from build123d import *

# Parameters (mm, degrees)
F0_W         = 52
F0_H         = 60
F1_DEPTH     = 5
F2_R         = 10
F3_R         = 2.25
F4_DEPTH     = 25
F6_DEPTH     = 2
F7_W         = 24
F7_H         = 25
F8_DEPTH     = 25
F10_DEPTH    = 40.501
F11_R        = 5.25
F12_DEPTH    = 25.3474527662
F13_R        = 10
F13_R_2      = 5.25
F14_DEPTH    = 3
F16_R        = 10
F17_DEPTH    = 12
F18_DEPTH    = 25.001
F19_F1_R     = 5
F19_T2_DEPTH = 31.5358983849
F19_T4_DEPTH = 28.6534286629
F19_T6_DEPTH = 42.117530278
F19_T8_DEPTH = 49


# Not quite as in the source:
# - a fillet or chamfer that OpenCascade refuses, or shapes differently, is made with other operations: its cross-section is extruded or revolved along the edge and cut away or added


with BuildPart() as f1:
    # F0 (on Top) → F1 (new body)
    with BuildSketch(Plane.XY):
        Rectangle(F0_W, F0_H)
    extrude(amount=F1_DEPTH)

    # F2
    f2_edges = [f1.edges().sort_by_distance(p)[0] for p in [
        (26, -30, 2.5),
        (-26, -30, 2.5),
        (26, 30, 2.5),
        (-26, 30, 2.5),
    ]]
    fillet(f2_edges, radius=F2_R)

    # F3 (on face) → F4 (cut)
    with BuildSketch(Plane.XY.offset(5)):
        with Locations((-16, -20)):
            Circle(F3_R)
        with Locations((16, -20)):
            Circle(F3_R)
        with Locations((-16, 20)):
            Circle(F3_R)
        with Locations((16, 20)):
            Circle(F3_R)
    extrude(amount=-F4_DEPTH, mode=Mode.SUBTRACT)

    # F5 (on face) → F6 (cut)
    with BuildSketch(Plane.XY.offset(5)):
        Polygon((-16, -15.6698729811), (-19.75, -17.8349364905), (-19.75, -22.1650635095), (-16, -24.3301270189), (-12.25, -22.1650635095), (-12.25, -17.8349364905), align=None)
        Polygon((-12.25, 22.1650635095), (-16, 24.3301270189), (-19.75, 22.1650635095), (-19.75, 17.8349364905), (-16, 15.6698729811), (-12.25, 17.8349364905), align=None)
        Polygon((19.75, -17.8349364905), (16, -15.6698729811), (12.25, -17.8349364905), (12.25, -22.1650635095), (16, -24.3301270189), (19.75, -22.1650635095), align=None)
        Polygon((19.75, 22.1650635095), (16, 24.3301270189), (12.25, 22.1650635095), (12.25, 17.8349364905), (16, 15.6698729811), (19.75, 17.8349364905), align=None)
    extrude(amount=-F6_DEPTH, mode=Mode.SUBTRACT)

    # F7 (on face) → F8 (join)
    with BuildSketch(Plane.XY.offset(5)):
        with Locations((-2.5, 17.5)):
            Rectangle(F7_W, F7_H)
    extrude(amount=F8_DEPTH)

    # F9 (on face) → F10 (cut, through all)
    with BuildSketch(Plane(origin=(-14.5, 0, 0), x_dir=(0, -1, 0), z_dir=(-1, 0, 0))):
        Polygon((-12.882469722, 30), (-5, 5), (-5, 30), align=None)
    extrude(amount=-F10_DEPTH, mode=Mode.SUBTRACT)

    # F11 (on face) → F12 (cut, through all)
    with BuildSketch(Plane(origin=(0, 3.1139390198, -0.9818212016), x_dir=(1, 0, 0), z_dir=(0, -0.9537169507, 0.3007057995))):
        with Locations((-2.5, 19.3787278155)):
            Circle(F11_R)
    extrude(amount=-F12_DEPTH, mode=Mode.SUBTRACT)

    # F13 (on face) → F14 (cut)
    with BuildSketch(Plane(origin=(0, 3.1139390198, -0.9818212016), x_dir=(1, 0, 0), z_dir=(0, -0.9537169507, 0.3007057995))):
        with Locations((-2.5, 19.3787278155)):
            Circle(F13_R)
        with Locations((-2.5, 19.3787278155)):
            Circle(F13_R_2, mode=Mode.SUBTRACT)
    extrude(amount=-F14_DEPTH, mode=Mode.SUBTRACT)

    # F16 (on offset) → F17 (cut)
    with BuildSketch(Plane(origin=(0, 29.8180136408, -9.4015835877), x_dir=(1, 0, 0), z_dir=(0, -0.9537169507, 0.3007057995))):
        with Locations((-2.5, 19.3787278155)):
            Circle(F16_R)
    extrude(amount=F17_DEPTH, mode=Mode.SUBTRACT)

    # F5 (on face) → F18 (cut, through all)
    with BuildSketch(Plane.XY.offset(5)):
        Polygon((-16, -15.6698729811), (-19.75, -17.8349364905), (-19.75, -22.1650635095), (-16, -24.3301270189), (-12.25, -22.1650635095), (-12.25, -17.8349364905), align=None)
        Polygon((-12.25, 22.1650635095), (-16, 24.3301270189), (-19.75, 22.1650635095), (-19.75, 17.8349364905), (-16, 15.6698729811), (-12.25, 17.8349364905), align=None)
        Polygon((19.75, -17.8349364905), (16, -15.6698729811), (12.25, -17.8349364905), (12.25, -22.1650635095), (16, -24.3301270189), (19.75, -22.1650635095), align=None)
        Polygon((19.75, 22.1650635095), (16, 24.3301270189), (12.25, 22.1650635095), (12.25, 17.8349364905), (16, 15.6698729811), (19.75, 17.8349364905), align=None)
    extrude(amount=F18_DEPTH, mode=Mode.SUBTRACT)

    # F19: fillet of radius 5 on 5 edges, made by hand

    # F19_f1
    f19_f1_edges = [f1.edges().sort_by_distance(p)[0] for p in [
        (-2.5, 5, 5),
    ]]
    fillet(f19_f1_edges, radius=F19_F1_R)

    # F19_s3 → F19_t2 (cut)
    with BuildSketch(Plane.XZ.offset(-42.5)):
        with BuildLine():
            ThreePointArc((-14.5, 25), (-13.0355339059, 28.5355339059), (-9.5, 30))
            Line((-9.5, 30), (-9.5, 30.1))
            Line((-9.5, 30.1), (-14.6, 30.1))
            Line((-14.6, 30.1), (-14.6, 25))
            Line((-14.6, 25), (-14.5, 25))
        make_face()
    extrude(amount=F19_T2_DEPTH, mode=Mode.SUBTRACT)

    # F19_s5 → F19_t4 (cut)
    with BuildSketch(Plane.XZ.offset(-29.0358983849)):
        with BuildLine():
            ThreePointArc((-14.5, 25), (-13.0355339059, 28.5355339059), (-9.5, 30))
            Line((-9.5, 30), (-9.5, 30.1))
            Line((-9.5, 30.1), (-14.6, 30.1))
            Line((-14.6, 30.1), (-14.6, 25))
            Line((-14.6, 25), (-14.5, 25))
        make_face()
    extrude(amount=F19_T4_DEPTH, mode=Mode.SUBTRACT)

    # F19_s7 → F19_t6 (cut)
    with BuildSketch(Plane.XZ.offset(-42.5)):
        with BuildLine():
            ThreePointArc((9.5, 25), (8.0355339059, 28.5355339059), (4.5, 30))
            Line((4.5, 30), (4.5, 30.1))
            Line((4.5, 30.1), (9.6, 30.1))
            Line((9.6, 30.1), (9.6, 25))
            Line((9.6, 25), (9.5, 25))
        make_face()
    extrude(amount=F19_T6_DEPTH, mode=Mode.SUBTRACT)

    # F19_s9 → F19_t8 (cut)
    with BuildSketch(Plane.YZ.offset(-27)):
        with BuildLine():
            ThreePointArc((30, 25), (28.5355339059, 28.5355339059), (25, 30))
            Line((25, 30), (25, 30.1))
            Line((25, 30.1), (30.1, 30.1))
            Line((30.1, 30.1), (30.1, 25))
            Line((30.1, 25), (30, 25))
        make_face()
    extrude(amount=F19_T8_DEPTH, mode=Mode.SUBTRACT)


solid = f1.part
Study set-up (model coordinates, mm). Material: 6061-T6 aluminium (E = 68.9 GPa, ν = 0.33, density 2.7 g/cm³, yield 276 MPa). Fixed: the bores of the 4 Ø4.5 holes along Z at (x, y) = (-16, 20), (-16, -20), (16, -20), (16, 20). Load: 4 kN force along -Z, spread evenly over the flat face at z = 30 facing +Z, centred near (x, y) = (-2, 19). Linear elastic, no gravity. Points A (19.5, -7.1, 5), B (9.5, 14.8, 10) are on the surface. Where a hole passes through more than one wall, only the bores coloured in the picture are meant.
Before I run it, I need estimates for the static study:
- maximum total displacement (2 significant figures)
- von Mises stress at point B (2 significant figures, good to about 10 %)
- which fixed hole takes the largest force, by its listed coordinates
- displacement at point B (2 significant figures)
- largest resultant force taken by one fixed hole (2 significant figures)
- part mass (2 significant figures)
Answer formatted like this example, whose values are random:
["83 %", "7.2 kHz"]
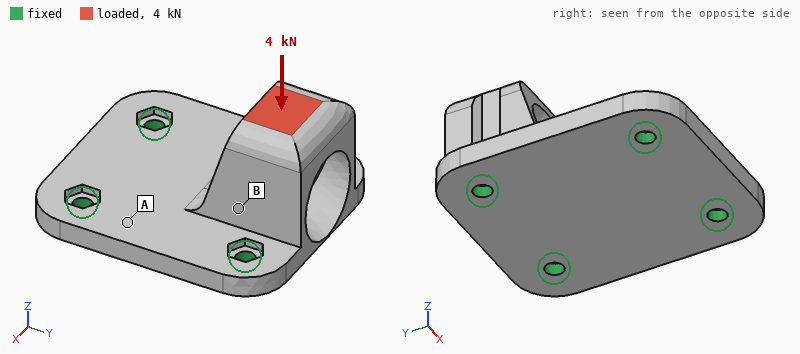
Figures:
["25 µm", "26 MPa", "(-16, 20)", "17 µm", "2.4 kN", "61 g"]
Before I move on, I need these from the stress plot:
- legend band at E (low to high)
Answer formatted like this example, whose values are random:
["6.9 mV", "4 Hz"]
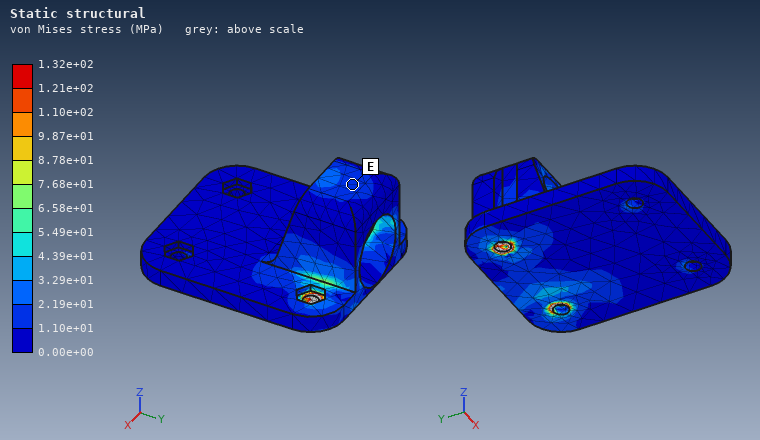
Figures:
["1.10e+01 to 2.19e+01 MPa"]
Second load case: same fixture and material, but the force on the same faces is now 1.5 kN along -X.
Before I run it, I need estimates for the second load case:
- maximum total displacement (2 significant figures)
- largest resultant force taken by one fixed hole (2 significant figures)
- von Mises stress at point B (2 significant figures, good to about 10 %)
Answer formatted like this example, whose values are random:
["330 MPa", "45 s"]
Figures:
["39 µm", "1.6 kN", "32 MPa"]
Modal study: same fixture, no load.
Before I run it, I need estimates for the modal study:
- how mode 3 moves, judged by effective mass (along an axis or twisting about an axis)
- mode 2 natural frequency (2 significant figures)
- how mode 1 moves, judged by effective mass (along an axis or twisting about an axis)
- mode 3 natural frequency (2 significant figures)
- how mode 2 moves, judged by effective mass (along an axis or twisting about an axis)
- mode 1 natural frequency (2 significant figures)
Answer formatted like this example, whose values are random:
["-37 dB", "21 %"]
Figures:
["along Z", "9800 Hz", "along Y", "13 kHz", "along X", "6100 Hz"]
